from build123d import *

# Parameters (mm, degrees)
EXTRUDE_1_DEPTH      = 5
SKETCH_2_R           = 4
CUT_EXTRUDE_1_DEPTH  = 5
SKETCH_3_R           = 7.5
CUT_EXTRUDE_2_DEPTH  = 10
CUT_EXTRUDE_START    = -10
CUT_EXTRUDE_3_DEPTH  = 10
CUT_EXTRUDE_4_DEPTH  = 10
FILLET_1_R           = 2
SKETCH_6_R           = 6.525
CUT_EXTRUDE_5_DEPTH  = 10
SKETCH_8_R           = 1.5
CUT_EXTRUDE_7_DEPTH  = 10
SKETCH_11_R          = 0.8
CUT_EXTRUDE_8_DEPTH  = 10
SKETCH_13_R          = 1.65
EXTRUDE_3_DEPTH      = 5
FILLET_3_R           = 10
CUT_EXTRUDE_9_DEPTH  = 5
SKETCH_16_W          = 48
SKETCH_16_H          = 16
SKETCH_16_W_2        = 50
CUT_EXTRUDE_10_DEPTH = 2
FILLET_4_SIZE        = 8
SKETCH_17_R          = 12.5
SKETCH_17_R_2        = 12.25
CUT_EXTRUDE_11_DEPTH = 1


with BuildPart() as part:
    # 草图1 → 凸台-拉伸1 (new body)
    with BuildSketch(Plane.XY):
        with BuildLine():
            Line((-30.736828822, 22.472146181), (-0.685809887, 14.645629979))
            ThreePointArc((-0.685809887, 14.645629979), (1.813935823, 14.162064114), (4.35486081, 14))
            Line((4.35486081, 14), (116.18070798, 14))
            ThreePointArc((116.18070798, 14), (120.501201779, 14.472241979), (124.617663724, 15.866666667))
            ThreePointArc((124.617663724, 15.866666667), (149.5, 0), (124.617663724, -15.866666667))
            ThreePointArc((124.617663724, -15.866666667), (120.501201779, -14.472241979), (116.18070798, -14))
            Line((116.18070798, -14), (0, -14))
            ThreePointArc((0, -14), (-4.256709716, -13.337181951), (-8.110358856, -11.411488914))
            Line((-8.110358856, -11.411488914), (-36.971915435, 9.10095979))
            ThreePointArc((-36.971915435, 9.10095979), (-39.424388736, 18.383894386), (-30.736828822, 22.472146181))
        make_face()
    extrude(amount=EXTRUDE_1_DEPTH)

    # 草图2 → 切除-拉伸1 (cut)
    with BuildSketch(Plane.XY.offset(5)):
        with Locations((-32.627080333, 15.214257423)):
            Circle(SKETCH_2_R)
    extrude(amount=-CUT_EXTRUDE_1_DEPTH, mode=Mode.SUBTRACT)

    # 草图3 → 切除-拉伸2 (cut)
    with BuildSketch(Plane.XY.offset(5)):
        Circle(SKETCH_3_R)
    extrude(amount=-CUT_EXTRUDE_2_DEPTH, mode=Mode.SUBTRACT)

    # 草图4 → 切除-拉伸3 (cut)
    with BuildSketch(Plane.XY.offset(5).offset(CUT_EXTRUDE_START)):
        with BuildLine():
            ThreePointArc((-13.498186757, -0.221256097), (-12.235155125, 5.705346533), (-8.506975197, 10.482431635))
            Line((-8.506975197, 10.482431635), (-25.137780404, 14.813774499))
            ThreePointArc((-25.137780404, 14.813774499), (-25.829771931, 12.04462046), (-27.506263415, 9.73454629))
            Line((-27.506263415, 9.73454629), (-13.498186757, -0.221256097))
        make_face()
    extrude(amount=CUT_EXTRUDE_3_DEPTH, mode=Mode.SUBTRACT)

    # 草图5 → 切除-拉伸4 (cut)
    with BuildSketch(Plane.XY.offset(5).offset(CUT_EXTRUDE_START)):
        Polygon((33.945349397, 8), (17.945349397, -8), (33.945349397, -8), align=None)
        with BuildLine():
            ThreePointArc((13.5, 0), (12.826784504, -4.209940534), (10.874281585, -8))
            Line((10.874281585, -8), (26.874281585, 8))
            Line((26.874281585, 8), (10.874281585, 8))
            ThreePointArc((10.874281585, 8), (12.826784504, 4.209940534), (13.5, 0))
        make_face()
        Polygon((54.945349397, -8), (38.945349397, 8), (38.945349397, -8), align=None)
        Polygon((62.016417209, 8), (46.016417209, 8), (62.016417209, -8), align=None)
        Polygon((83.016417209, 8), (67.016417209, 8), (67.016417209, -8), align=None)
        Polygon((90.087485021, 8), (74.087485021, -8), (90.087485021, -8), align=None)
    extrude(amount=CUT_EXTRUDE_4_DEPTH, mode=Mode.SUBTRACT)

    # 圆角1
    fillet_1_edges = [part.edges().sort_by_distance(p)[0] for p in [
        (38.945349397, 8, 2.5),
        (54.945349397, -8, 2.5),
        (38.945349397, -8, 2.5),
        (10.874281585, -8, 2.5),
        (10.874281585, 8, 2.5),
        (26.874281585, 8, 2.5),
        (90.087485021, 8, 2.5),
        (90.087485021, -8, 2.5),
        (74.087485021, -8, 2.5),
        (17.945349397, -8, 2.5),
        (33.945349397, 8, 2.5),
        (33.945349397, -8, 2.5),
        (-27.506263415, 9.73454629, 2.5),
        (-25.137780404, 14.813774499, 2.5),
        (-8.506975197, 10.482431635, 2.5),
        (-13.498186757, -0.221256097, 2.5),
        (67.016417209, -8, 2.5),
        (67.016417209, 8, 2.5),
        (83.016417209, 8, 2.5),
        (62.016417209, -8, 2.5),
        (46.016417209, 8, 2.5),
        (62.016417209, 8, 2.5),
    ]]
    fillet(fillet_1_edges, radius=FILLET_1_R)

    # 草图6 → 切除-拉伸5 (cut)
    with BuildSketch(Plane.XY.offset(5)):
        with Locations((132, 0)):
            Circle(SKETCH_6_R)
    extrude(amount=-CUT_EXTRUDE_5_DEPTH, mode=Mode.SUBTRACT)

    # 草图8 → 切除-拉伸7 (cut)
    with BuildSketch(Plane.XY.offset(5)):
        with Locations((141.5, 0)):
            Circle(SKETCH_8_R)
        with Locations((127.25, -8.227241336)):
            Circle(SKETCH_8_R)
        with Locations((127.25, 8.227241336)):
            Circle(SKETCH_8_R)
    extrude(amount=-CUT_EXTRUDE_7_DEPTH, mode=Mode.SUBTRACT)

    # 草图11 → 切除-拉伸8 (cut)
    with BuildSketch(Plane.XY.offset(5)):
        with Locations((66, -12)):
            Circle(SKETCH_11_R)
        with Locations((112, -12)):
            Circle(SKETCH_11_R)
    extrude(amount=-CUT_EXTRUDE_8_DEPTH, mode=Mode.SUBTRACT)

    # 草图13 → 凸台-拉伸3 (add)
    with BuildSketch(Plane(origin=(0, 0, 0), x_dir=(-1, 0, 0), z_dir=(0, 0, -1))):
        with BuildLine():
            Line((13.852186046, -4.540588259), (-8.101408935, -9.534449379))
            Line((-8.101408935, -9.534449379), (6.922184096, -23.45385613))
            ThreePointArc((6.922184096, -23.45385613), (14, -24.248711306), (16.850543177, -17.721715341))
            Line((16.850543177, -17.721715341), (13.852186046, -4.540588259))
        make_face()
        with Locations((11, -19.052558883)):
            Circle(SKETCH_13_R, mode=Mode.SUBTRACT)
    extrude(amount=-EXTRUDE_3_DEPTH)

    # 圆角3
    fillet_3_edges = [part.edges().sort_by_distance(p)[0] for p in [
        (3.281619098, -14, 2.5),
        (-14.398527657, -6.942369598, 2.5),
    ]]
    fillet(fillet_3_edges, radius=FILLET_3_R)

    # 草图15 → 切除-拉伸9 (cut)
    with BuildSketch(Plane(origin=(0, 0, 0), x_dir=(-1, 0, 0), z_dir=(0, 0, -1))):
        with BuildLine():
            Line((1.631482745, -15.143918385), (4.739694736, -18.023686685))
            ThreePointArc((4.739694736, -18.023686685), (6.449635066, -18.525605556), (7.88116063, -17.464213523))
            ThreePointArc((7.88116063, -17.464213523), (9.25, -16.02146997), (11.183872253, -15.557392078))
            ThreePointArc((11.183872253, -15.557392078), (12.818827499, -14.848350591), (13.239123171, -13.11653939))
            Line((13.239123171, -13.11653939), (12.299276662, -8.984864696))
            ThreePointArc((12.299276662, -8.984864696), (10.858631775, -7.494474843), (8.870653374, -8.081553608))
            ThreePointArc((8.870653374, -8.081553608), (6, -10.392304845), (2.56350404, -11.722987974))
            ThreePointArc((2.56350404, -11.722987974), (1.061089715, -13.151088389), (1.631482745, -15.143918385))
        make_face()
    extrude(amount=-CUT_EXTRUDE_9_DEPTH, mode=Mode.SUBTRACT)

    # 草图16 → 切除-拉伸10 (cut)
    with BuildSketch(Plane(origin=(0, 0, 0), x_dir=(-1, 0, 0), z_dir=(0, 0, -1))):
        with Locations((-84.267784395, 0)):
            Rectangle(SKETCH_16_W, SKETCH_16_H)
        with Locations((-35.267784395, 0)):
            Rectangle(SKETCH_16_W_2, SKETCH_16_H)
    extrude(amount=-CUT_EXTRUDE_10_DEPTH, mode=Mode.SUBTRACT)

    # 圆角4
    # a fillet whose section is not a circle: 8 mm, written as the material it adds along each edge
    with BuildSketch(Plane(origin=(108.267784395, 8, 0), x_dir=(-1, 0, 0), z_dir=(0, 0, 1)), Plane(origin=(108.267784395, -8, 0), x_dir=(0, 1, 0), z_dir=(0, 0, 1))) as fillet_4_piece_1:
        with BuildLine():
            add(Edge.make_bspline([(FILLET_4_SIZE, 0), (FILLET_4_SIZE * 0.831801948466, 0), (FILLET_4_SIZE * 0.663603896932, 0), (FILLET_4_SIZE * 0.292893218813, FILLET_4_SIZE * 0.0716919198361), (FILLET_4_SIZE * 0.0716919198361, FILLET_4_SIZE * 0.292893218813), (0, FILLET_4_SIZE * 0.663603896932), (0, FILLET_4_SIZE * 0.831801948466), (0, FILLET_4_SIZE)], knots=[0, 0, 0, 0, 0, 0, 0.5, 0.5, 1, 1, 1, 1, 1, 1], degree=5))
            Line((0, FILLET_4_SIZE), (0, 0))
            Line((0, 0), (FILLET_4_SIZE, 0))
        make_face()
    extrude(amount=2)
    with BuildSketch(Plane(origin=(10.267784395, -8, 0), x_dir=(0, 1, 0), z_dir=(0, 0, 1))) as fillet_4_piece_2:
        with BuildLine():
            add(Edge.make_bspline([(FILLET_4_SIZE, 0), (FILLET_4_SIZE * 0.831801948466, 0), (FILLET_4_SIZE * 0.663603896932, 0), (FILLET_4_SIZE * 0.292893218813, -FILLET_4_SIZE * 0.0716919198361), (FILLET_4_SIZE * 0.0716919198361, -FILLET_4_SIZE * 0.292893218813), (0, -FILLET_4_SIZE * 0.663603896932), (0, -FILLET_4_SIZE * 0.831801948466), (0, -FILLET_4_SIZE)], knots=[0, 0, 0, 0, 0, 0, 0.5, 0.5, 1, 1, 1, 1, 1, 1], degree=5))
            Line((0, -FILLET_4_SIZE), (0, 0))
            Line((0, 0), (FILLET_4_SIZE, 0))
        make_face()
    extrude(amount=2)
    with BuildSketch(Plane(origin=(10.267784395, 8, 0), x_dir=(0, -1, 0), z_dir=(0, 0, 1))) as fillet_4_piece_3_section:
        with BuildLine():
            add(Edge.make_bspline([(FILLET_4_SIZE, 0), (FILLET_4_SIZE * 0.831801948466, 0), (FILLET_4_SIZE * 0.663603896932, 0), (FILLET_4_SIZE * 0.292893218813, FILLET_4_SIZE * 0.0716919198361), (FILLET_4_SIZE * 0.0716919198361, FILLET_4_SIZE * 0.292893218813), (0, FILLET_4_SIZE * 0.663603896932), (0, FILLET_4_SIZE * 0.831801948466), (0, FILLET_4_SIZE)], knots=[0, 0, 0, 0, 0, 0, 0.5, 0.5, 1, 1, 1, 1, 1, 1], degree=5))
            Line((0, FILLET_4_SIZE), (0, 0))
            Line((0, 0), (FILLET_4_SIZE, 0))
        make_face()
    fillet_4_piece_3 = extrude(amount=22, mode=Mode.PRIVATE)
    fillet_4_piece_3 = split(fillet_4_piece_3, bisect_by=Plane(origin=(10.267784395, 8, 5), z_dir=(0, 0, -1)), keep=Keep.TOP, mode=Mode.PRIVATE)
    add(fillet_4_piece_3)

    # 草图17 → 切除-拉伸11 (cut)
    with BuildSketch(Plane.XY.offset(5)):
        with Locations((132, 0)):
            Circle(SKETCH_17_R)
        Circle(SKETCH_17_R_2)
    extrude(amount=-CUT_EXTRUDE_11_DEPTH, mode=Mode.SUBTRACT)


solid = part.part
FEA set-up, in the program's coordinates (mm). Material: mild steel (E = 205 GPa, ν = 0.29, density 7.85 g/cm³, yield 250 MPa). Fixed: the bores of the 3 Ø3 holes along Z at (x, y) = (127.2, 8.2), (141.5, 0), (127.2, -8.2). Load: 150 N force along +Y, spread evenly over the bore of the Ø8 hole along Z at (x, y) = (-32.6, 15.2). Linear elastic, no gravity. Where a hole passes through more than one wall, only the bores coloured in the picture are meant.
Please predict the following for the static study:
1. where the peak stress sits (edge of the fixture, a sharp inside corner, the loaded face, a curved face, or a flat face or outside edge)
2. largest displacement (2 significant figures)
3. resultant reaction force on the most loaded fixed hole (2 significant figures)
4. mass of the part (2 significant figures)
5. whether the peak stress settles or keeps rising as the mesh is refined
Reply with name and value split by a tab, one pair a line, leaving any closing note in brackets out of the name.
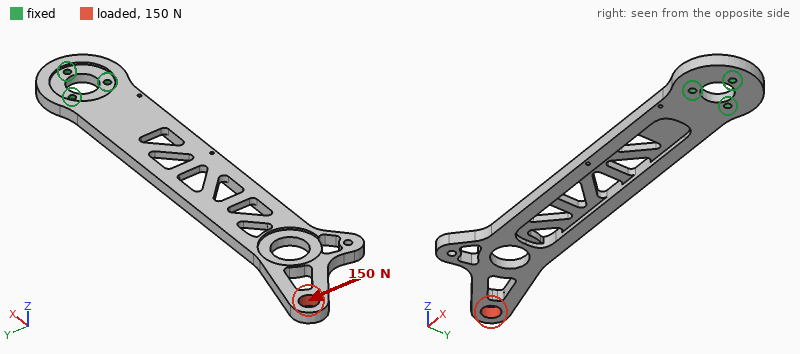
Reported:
where the peak stress sits	edge of the fixture
largest displacement	0.16 mm
resultant reaction force on the most loaded fixed hole	1.2 kN
mass of the part	140 g
whether the peak stress settles or keeps rising as the mesh is refined	keeps rising
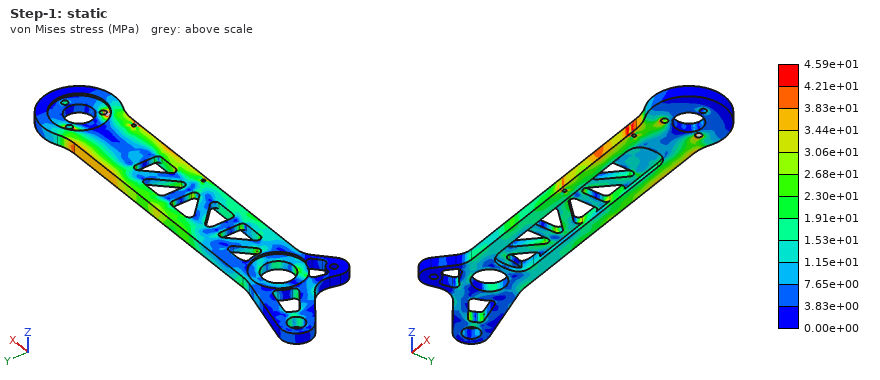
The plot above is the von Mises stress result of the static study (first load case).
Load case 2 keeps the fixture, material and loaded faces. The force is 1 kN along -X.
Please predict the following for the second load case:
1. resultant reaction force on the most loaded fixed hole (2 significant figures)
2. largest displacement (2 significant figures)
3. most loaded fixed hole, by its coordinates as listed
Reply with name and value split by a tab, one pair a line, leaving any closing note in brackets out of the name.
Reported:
resultant reaction force on the most loaded fixed hole	1.2 kN
largest displacement	0.15 mm
most loaded fixed hole, by its coordinates as listed	(127.2, 8.2)
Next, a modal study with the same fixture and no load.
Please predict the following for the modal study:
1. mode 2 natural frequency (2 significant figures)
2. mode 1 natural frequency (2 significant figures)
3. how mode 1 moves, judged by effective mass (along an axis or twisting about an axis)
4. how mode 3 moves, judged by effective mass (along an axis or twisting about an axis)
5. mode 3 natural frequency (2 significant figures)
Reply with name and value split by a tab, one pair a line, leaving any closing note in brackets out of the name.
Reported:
mode 2 natural frequency	820 Hz
mode 1 natural frequency	150 Hz
how mode 1 moves, judged by effective mass	along Z
how mode 3 moves, judged by effective mass	along Y
mode 3 natural frequency	920 Hz
